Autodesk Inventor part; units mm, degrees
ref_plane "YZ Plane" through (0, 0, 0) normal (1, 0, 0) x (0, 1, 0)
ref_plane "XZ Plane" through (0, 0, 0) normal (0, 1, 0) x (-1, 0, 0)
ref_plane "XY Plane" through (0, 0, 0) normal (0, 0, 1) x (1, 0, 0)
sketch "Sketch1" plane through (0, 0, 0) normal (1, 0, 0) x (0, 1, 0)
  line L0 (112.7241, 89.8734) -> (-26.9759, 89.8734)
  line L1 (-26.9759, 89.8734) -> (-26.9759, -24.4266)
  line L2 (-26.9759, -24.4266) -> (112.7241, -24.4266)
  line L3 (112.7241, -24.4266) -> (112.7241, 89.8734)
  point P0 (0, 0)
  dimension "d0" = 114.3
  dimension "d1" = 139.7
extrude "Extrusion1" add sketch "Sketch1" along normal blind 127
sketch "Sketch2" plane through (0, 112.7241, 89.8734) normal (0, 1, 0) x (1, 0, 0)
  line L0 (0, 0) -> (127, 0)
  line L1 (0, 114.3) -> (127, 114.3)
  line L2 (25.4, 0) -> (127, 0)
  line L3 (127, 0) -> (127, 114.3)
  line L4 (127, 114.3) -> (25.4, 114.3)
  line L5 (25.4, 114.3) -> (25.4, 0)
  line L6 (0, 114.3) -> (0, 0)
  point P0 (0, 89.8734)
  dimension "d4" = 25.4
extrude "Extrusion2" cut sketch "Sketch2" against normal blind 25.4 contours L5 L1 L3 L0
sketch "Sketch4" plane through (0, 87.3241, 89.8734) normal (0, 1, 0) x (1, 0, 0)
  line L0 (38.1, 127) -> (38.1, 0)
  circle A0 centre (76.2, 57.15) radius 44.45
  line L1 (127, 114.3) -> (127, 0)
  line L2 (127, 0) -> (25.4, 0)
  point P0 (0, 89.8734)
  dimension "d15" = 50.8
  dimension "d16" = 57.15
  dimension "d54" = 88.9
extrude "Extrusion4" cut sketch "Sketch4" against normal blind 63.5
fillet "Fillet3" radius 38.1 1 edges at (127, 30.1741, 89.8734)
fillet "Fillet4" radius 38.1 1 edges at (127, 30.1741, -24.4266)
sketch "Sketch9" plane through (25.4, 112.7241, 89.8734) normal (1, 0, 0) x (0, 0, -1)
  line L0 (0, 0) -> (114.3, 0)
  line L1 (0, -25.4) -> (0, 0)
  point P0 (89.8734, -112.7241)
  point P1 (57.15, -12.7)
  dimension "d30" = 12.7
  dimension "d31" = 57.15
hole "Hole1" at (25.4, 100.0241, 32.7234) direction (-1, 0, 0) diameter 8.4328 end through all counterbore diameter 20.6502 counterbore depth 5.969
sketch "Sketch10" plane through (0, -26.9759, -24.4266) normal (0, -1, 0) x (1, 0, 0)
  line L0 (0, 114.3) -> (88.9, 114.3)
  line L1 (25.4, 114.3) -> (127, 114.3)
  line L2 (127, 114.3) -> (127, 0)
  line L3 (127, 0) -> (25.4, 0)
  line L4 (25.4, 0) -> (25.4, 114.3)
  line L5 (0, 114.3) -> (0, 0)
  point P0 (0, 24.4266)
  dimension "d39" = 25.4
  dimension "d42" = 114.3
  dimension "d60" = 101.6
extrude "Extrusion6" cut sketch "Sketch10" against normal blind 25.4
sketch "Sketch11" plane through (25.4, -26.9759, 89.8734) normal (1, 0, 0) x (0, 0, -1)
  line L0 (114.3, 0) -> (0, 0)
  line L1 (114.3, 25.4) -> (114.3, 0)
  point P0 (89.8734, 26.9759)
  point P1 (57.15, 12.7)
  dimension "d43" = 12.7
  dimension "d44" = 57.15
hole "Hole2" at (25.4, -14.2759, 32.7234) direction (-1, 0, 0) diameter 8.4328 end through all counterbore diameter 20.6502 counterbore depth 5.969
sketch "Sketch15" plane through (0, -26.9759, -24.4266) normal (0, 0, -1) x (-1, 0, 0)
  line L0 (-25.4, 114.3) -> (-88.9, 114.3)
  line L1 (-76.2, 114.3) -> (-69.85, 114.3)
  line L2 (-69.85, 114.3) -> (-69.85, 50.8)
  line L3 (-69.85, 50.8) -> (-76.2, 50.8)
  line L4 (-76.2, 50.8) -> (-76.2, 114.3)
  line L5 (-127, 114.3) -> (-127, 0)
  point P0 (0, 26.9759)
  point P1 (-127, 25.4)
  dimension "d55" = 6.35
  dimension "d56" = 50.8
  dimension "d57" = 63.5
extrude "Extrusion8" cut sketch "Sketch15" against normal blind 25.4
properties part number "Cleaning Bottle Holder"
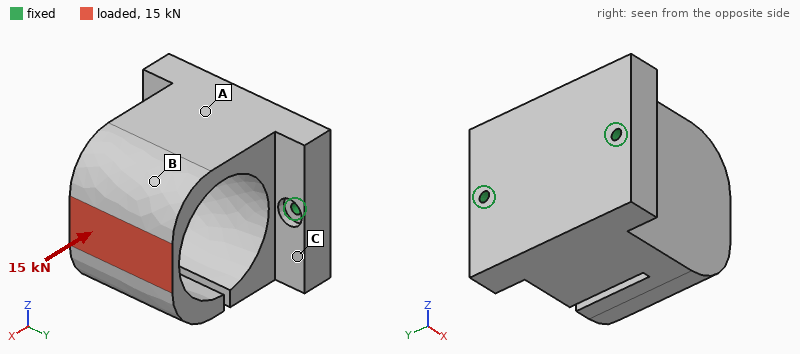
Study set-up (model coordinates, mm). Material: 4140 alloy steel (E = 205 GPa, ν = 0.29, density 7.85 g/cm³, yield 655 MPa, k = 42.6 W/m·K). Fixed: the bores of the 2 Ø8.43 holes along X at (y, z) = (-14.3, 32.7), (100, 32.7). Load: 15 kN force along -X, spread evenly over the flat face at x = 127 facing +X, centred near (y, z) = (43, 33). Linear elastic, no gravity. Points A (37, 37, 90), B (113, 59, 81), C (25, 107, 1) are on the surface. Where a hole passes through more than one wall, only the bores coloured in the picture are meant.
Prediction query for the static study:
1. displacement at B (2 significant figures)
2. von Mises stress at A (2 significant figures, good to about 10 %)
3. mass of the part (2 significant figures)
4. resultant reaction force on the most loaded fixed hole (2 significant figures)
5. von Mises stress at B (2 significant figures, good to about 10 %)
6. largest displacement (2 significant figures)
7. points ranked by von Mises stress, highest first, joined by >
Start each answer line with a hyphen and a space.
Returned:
- 17 µm
- 13 MPa
- 7.7 kg
- 8.2 kN
- 22 MPa
- 73 µm
- B > A > C
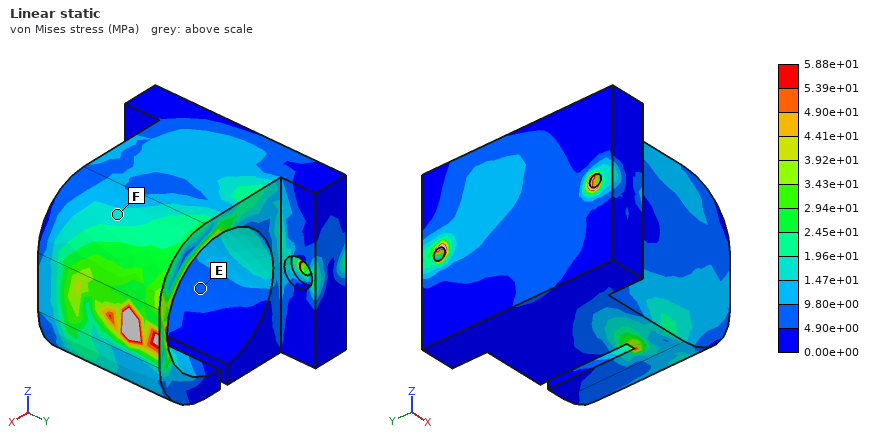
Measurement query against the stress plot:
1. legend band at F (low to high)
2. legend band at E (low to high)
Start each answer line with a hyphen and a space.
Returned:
- 1.47e+01 to 1.96e+01 MPa
- 4.90e+00 to 9.80e+00 MPa
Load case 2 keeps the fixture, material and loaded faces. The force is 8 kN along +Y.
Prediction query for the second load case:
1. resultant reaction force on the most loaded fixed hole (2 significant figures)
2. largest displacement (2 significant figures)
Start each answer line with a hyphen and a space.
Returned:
- 9.7 kN
- 59 µm
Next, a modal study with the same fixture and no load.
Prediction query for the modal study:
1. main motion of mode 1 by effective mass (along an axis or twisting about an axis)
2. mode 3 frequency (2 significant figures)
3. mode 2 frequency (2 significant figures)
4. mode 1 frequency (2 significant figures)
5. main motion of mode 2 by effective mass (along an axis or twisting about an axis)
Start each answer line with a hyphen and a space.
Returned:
- along Z
- 3000 Hz
- 1900 Hz
- 840 Hz
- along Y
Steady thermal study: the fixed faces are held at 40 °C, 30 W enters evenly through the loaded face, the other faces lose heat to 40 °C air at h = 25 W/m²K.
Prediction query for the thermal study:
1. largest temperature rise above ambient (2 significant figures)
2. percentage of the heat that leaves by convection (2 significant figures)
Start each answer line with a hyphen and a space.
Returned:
- 24 K
- 57 %
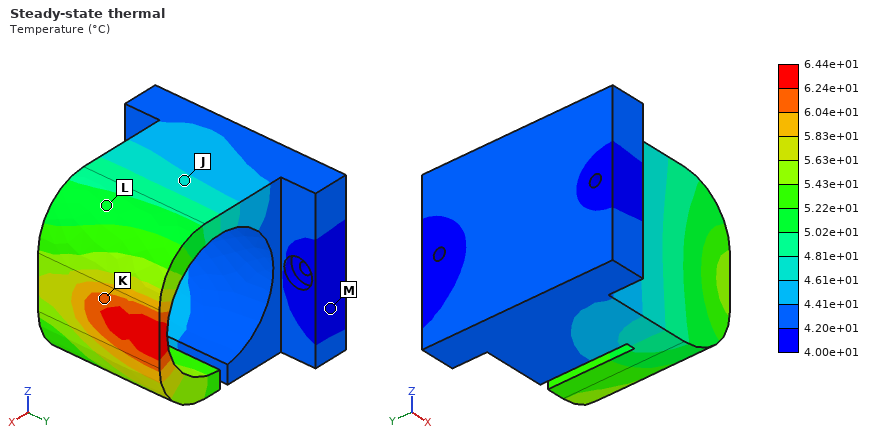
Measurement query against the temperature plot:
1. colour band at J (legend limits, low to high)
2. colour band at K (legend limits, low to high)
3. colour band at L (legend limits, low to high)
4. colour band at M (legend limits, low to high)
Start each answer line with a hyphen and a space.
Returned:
- 4.61e+01 to 4.81e+01 °C
- 6.04e+01 to 6.24e+01 °C
- 5.02e+01 to 5.22e+01 °C
- 4.00e+01 to 4.20e+01 °C
